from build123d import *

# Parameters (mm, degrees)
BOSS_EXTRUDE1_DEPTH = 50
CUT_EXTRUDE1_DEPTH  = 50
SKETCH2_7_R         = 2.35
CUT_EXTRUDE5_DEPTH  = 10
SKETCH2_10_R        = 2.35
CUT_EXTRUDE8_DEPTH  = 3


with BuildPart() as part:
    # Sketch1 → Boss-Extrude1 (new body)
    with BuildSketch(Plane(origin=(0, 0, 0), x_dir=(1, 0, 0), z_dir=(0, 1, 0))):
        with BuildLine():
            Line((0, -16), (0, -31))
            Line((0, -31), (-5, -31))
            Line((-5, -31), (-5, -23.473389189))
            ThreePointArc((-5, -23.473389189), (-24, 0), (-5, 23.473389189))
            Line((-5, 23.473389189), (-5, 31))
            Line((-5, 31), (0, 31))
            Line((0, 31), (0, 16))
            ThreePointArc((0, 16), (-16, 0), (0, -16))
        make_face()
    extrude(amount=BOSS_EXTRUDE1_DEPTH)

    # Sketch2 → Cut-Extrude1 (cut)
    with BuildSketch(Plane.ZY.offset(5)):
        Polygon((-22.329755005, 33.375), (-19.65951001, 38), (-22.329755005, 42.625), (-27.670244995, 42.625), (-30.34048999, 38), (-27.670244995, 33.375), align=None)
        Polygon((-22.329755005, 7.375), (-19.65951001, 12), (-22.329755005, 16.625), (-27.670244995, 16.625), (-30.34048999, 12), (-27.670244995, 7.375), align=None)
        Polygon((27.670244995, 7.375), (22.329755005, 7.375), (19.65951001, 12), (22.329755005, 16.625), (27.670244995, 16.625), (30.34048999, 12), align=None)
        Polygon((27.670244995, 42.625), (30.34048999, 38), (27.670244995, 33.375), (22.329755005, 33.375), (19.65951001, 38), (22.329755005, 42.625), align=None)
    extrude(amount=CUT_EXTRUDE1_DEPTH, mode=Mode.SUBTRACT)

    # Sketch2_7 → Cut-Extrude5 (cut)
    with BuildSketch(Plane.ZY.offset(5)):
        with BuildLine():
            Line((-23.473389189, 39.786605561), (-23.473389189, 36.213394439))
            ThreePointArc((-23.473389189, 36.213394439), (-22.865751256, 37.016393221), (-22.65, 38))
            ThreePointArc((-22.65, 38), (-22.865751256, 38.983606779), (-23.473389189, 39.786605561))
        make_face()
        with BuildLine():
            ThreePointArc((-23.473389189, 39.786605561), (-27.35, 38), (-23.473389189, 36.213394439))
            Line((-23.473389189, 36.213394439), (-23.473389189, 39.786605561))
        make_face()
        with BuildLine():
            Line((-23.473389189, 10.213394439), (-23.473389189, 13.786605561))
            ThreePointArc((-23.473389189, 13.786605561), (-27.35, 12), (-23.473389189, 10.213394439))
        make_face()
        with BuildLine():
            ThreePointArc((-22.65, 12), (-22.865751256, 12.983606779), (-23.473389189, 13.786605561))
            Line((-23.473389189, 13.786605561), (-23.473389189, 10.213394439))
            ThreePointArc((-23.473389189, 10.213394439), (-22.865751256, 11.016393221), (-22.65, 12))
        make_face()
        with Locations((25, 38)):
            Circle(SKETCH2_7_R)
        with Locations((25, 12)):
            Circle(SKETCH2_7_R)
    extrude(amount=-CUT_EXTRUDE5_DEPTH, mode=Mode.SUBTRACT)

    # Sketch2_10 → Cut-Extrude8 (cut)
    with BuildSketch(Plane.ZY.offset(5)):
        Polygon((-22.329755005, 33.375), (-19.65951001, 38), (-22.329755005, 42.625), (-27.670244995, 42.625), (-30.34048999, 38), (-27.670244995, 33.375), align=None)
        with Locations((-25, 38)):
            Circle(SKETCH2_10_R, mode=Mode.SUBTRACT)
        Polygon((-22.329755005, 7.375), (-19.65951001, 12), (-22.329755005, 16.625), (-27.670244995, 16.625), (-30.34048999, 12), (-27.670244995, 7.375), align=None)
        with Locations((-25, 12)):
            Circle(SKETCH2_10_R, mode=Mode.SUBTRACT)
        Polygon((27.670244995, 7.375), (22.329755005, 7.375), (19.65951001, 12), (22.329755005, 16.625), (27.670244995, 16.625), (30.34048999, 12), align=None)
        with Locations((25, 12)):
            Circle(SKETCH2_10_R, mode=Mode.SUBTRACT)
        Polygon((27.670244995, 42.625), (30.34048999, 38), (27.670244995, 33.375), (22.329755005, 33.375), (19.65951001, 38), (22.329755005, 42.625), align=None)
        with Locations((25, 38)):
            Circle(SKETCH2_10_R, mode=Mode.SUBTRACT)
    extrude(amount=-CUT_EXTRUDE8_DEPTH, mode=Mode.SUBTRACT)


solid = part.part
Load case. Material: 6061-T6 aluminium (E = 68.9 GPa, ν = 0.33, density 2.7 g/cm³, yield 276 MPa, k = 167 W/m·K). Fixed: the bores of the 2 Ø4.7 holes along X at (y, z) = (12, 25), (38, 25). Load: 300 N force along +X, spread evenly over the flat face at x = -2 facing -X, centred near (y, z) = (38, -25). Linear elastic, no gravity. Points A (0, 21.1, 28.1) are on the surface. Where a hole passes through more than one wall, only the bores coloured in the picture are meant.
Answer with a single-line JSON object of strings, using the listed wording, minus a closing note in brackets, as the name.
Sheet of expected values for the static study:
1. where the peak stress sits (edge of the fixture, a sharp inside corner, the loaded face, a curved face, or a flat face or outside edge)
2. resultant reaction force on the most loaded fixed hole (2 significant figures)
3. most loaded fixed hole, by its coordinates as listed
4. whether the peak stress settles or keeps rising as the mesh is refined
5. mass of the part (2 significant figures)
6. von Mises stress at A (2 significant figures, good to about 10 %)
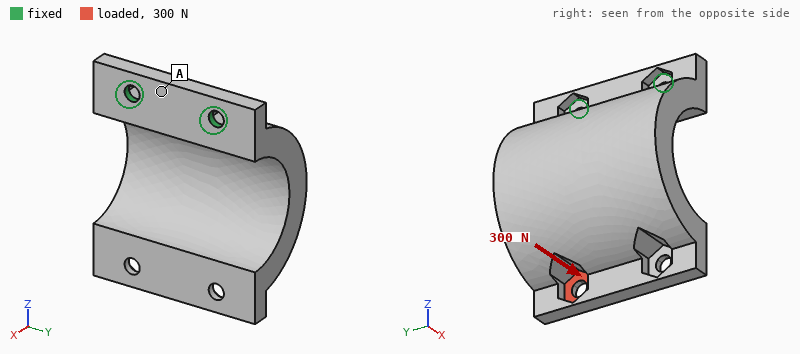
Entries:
{"where the peak stress sits": "edge of the fixture", "resultant reaction force on the most loaded fixed hole": "290 N", "most loaded fixed hole, by its coordinates as listed": "(38, 25)", "whether the peak stress settles or keeps rising as the mesh is refined": "keeps rising", "mass of the part": "74 g", "von Mises stress at A": "40 MPa"}
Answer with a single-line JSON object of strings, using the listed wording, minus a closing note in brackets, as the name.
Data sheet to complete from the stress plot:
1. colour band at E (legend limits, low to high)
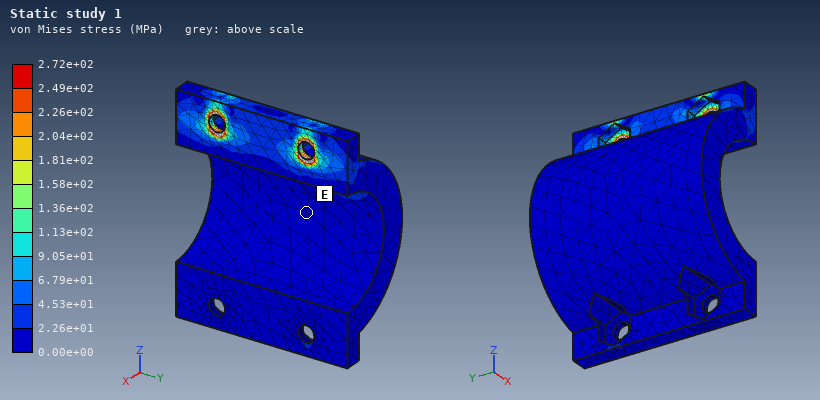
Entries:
{"colour band at E": "0.00e+00 to 2.26e+01 MPa"}
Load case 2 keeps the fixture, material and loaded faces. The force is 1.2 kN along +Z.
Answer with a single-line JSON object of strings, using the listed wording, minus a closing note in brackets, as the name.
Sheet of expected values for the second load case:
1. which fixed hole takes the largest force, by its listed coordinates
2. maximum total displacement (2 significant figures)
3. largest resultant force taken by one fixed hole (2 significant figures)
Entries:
{"which fixed hole takes the largest force, by its listed coordinates": "(38, 25)", "maximum total displacement": "0.20 mm", "largest resultant force taken by one fixed hole": "1.1 kN"}
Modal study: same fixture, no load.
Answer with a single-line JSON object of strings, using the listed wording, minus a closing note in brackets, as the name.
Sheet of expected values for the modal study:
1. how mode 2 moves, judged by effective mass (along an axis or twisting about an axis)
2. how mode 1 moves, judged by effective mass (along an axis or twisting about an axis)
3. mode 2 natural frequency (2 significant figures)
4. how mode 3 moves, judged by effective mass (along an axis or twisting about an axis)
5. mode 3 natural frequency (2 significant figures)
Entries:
{"how mode 2 moves, judged by effective mass": "along Y", "how mode 1 moves, judged by effective mass": "along X", "mode 2 natural frequency": "2200 Hz", "how mode 3 moves, judged by effective mass": "along Z", "mode 3 natural frequency": "4100 Hz"}
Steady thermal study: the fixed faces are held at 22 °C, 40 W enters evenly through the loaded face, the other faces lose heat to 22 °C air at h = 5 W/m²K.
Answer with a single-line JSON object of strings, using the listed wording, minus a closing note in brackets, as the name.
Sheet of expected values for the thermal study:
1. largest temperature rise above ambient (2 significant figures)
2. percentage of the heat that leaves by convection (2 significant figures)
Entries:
{"largest temperature rise above ambient": "78 K", "percentage of the heat that leaves by convection": "3.7 %"}
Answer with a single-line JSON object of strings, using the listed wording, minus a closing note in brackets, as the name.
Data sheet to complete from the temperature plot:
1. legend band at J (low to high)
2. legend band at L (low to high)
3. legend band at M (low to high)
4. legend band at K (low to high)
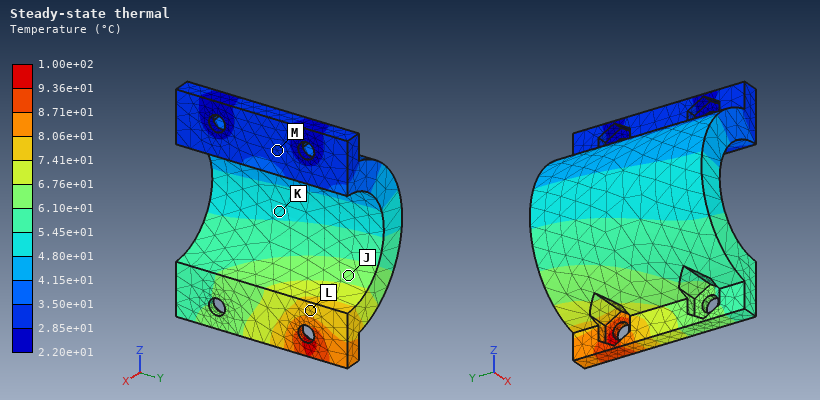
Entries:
{"legend band at J": "6.10e+01 to 6.76e+01 °C", "legend band at L": "7.41e+01 to 8.06e+01 °C", "legend band at M": "2.85e+01 to 3.50e+01 °C", "legend band at K": "4.80e+01 to 5.45e+01 °C"}
